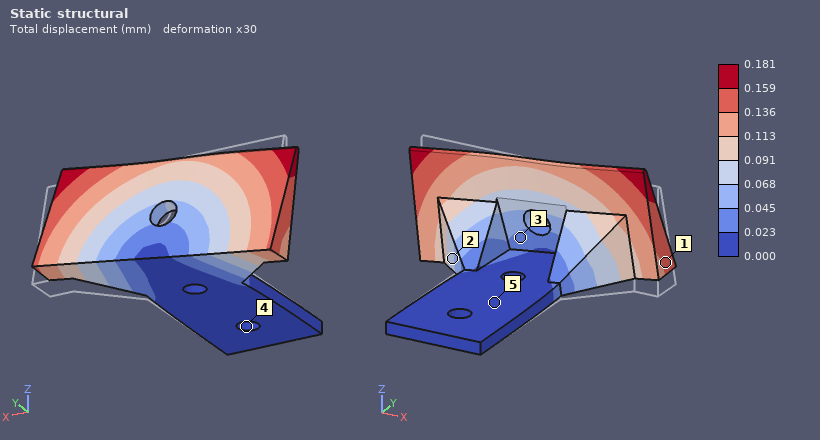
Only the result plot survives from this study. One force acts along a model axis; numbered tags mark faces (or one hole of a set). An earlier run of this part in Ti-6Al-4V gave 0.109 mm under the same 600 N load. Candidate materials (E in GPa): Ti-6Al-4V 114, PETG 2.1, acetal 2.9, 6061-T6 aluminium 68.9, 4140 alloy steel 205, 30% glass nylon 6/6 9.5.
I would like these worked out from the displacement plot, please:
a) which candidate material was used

6061-T6 aluminium
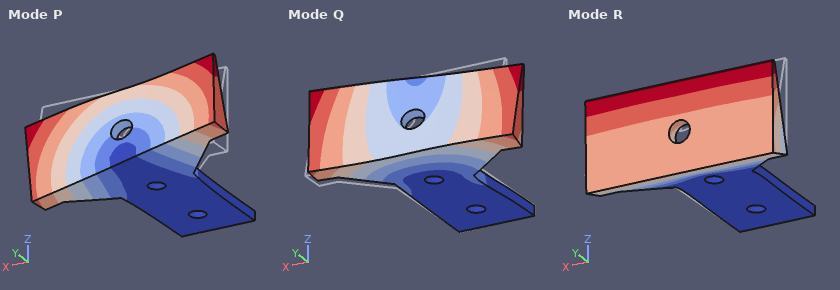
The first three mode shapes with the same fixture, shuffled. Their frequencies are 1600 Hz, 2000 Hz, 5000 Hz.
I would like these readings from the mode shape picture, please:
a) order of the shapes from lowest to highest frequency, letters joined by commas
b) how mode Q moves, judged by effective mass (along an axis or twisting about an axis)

P, R, Q
along X
